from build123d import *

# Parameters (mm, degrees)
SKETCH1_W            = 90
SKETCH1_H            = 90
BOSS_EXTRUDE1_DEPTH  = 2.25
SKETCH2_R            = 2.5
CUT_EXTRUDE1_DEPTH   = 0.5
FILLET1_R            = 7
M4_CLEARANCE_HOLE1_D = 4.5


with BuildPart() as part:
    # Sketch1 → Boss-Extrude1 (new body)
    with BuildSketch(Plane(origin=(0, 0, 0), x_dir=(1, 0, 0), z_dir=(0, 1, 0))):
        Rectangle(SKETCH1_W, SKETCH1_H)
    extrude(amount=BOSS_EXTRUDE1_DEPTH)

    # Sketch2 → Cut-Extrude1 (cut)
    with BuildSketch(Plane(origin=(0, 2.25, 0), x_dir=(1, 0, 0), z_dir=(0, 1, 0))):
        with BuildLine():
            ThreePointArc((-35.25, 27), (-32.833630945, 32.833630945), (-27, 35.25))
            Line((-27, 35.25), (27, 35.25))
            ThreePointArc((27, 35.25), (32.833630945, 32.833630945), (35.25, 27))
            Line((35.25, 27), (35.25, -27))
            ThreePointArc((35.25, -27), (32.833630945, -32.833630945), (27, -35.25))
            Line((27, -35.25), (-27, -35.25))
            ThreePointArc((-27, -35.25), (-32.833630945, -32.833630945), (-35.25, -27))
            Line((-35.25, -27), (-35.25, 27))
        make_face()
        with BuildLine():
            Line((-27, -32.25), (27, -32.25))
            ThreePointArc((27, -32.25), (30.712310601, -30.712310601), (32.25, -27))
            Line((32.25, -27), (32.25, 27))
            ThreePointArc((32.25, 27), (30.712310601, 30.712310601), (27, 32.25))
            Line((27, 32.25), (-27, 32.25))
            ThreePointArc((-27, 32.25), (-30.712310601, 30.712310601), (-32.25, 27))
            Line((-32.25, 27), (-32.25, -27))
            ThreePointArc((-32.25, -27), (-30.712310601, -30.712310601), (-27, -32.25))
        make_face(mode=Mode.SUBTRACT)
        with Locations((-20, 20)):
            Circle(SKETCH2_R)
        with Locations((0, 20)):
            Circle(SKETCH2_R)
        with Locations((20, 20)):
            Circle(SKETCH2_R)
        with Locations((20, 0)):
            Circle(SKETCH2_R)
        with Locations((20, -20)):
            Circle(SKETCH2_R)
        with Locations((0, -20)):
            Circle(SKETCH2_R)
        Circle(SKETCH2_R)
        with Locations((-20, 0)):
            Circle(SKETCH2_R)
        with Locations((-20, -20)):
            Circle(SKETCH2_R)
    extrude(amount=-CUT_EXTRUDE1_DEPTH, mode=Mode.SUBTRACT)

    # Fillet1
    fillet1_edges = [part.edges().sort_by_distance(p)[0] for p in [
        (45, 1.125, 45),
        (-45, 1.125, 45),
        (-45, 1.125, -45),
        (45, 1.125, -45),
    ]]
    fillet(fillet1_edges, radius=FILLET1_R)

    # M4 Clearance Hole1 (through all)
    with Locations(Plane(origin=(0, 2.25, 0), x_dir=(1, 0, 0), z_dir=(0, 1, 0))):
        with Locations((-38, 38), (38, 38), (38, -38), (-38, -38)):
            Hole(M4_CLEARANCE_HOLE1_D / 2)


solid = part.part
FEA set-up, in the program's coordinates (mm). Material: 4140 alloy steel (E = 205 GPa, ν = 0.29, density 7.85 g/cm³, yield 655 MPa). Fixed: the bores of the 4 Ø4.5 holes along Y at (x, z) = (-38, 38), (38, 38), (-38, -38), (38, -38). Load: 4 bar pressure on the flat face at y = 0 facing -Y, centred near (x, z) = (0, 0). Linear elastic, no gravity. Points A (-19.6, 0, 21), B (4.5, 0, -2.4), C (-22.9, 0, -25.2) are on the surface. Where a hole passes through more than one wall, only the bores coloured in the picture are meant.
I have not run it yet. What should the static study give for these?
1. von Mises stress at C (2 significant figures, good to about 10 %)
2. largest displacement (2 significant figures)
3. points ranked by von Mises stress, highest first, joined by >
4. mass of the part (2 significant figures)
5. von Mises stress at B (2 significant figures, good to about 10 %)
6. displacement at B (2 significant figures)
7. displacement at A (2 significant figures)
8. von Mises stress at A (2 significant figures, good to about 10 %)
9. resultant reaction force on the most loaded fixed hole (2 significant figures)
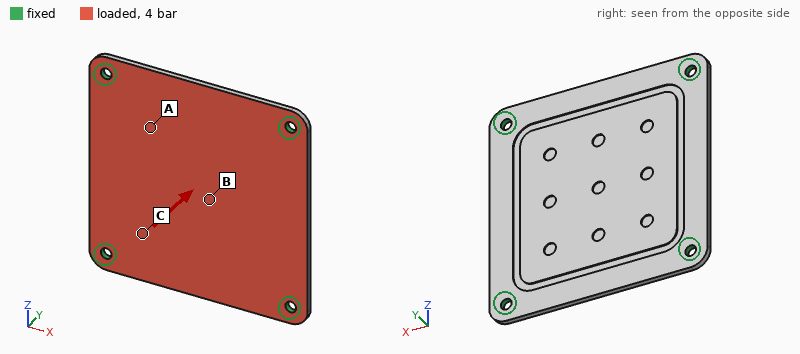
49 MPa
0.49 mm
B > A > C
140 g
150 MPa
0.48 mm
0.30 mm
87 MPa
800 N
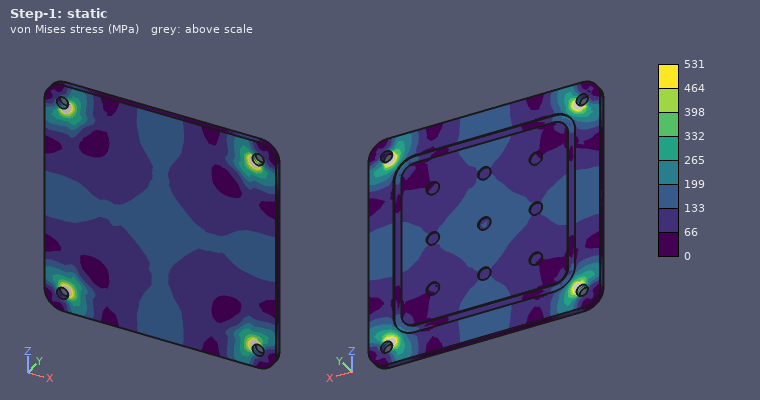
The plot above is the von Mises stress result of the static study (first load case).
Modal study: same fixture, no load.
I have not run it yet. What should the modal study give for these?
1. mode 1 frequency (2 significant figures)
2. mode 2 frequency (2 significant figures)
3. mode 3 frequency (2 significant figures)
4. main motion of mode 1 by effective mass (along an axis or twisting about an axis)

1300 Hz
2300 Hz
2300 Hz
along Y
